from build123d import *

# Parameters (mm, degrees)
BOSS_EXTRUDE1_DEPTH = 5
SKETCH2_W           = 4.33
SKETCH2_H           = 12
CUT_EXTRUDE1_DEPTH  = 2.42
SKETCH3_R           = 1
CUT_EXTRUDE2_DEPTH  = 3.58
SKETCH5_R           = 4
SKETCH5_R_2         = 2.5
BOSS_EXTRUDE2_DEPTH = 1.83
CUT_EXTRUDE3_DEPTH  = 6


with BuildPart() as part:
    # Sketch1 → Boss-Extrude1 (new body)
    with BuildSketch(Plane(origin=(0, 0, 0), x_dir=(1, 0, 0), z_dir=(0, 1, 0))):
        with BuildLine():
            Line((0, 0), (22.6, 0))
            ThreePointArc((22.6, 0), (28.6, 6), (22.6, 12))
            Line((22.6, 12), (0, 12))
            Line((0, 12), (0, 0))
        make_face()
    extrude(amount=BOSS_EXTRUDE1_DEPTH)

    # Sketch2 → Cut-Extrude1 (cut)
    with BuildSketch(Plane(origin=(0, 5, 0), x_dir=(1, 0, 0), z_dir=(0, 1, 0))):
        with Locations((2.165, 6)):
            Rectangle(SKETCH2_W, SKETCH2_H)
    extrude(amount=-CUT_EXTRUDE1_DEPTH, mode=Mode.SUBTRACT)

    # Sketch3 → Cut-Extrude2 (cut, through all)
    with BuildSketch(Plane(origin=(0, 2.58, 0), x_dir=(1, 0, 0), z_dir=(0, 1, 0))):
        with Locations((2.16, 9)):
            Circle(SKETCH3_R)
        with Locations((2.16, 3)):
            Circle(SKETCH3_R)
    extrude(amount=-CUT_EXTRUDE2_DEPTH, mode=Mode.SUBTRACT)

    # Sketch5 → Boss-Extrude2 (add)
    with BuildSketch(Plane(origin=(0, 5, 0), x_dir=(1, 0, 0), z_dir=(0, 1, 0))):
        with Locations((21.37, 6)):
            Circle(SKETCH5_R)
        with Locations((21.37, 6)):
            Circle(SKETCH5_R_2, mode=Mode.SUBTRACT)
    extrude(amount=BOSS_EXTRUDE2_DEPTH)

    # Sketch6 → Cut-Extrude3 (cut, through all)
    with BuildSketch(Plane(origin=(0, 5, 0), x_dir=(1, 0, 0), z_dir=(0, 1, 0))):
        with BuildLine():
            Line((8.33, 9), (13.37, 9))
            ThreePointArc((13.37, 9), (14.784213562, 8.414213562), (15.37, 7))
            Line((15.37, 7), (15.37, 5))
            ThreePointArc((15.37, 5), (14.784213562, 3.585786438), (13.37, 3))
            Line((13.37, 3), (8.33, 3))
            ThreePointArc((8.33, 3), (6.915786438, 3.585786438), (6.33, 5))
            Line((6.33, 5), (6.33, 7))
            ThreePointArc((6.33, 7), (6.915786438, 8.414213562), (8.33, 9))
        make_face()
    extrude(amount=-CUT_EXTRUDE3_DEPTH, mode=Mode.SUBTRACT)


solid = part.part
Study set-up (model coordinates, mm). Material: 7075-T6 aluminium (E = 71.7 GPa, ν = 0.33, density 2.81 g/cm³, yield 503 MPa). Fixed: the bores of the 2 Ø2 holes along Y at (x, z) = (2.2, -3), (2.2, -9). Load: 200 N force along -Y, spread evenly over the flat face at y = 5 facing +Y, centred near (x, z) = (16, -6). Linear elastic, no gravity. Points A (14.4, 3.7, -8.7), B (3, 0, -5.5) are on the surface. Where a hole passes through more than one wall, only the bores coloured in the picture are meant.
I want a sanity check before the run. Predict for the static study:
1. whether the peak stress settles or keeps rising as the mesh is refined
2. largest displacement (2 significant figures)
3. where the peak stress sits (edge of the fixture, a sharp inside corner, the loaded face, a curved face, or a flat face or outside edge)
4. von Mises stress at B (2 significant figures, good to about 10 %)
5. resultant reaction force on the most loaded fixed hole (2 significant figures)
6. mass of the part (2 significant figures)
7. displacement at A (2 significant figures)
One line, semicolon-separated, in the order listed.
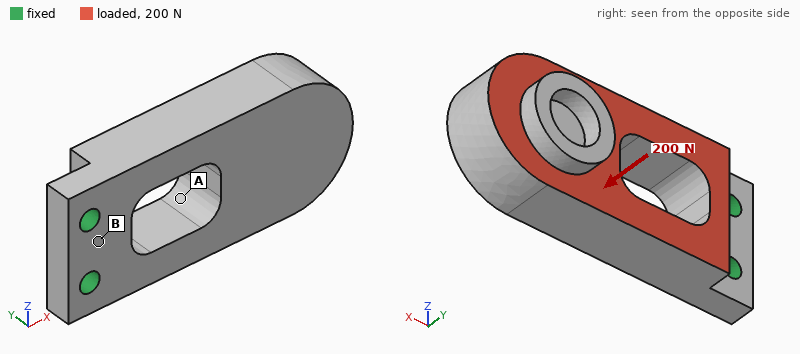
keeps rising; 0.21 mm; edge of the fixture; 87 MPa; 100 N; 3.6 g; 0.080 mm
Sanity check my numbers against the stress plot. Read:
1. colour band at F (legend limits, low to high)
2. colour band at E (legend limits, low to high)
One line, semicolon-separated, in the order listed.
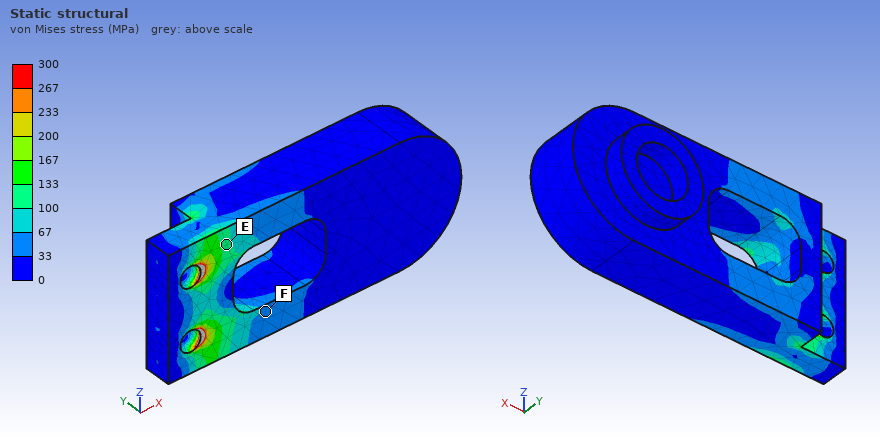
33 to 67 MPa; 100 to 133 MPa
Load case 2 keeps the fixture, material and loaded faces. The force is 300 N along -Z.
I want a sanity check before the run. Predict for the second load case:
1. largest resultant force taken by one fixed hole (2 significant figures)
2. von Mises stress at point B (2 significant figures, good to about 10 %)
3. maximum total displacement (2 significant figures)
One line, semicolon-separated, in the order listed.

540 N; 19 MPa; 48 µm
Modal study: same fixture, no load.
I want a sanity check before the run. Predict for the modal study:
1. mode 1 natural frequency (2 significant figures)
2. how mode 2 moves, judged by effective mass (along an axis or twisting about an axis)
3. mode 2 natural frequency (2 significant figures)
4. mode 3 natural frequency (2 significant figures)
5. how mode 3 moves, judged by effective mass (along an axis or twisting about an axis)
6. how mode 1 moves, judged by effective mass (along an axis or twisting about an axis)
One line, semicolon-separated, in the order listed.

3100 Hz; along Z; 7500 Hz; 14 kHz; twisting about X; along Y
